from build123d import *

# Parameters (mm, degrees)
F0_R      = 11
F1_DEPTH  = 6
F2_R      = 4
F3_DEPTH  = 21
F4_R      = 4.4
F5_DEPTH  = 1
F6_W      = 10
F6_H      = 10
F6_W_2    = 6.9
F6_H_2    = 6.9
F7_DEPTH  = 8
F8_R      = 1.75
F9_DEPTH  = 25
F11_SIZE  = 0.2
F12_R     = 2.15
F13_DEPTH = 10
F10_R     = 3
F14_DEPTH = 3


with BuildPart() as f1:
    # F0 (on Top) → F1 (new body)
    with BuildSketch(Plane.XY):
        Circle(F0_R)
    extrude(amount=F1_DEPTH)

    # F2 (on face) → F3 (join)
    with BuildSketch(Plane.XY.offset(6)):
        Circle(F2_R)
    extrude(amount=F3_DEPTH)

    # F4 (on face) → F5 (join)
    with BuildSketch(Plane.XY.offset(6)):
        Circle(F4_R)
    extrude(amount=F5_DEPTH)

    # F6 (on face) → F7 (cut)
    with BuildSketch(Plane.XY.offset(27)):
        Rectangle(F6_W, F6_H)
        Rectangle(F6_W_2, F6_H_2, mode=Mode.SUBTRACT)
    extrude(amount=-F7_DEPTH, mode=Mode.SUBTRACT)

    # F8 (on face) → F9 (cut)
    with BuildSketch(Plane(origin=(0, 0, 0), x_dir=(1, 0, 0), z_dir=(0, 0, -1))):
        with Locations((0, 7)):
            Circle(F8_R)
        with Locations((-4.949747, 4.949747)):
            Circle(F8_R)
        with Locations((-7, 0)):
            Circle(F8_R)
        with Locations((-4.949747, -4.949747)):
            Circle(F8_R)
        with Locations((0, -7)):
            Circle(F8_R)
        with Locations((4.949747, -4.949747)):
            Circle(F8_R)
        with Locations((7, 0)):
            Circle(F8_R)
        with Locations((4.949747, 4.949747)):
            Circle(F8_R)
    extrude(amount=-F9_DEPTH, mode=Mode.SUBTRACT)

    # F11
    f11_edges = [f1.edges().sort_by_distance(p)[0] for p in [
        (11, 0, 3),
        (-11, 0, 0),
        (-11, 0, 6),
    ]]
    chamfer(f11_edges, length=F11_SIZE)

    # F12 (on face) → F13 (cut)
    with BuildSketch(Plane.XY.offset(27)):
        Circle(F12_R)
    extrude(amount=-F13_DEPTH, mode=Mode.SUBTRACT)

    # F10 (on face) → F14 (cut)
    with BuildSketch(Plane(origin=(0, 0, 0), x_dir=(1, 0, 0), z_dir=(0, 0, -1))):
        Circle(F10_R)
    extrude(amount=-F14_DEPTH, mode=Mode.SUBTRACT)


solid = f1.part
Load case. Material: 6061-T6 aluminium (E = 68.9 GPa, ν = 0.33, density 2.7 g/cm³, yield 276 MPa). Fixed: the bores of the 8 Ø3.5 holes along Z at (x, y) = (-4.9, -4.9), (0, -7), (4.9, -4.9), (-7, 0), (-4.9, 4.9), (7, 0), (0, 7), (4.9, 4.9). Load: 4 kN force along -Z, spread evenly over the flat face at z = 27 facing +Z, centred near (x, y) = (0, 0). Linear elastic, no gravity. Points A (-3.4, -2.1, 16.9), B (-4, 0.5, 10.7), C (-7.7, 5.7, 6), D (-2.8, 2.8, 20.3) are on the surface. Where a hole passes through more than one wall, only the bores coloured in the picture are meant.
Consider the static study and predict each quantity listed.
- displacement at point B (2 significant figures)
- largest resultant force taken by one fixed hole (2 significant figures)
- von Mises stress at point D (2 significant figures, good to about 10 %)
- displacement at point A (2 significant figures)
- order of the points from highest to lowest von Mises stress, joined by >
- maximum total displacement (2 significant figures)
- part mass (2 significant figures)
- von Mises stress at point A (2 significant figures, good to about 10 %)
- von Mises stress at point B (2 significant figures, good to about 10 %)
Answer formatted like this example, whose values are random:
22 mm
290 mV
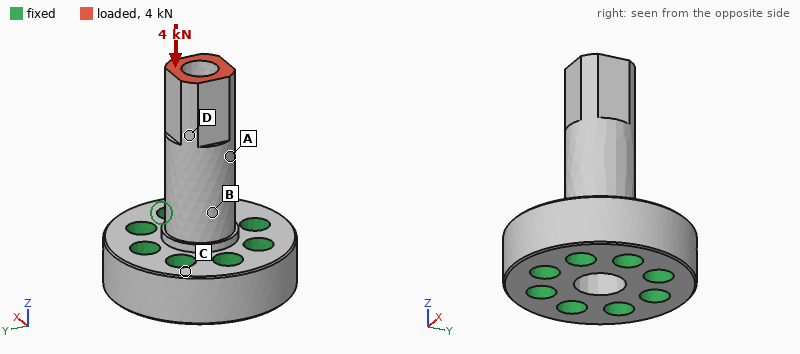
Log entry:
8.5 µm
630 N
130 MPa
17 µm
D > A > B > C
35 µm
7.0 g
100 MPa
80 MPa
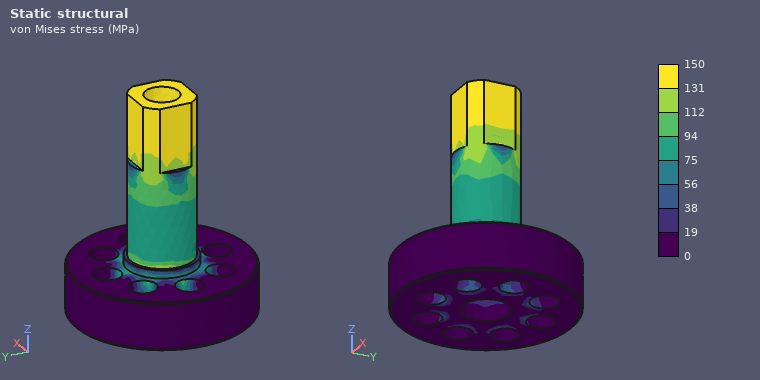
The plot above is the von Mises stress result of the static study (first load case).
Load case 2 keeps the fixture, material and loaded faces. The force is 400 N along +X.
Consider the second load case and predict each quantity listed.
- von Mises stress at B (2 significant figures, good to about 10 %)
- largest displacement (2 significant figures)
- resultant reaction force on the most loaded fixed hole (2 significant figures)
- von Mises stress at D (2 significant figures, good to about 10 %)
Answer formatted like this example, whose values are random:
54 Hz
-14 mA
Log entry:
130 MPa
0.12 mm
470 N
55 MPa
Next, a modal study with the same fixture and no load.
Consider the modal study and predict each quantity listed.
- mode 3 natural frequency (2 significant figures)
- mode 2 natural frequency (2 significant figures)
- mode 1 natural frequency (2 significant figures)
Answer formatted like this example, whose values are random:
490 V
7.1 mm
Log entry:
39 kHz
14 kHz
14 kHz
